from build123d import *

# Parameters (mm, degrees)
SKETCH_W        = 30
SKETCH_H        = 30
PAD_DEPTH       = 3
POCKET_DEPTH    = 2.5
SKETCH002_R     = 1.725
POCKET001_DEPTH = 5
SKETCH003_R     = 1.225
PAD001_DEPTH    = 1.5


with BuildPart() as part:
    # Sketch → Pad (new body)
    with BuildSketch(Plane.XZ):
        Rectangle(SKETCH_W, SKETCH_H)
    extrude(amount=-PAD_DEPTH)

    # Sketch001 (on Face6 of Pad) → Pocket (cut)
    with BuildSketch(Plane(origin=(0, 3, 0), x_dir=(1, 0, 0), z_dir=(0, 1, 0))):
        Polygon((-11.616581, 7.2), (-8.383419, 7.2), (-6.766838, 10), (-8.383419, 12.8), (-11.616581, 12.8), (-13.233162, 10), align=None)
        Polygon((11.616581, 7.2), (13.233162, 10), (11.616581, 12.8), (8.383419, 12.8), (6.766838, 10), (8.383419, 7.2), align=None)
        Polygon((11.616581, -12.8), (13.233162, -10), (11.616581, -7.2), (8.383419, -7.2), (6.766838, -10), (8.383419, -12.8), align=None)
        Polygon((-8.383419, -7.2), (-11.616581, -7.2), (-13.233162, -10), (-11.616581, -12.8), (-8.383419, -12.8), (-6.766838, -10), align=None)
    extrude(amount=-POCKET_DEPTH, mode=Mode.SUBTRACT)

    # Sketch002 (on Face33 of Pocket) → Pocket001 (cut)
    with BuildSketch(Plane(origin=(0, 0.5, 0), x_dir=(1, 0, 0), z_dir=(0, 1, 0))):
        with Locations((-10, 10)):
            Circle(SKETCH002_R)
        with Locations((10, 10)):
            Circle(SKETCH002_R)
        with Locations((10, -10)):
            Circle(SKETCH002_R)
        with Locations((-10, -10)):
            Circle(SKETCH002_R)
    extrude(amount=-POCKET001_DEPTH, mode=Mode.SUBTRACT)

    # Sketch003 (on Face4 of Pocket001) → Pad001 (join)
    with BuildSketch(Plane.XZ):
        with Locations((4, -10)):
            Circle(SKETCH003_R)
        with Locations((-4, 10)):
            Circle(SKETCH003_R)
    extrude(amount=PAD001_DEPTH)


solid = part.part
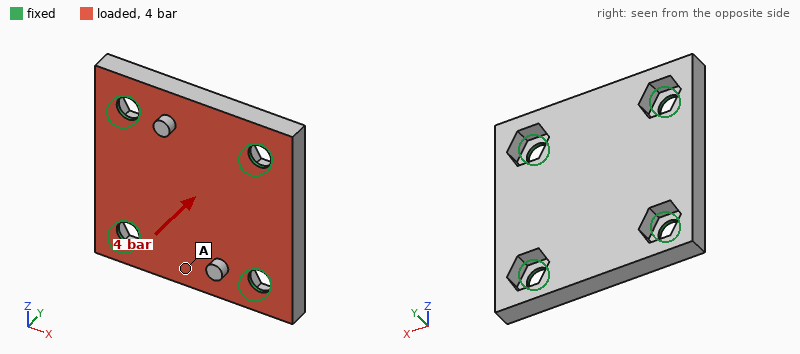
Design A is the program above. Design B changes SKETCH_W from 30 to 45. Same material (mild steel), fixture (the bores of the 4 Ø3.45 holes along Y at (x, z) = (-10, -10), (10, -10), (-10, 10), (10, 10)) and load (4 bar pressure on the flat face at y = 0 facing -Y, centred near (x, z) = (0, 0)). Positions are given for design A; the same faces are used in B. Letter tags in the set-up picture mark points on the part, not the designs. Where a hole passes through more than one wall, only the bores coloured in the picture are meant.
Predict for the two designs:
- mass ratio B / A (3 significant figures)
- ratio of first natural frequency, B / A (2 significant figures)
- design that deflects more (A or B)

1.56
0.51
B
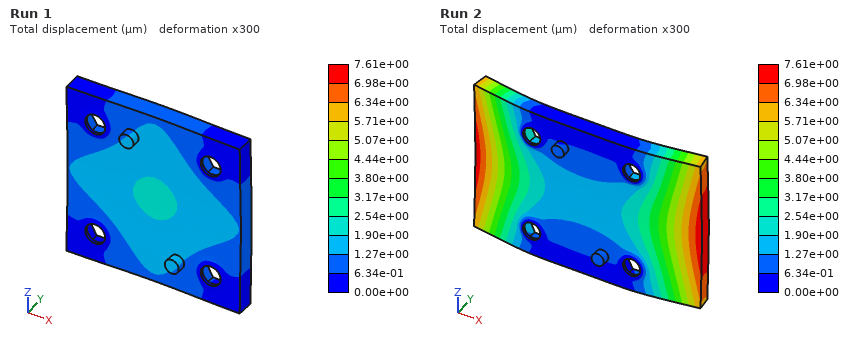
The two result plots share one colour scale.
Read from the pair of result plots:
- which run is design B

Run 2
